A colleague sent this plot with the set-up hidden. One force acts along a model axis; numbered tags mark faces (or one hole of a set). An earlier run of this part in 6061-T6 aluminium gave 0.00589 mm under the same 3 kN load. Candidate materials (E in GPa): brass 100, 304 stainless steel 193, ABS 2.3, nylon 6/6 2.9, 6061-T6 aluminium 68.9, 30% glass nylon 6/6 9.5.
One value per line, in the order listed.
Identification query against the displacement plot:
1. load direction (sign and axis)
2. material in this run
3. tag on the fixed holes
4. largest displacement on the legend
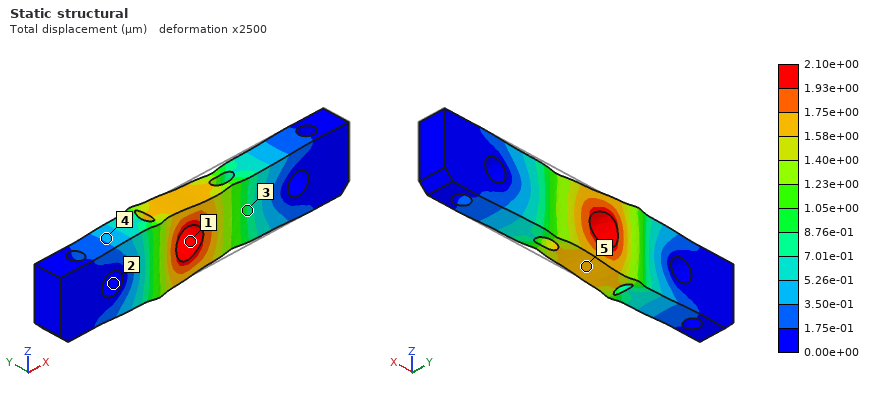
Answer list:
-X
304 stainless steel
2
2.10e+00 µm
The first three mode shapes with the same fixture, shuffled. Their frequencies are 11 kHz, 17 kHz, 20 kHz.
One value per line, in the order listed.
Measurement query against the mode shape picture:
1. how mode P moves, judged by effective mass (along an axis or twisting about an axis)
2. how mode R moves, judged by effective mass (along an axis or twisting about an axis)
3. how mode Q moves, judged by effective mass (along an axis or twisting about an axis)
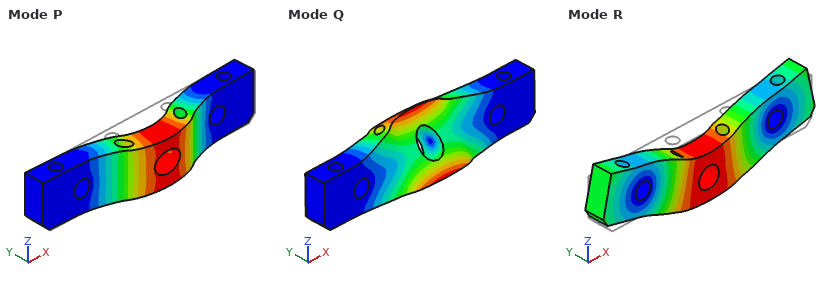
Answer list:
along Y
along Z
twisting about X
